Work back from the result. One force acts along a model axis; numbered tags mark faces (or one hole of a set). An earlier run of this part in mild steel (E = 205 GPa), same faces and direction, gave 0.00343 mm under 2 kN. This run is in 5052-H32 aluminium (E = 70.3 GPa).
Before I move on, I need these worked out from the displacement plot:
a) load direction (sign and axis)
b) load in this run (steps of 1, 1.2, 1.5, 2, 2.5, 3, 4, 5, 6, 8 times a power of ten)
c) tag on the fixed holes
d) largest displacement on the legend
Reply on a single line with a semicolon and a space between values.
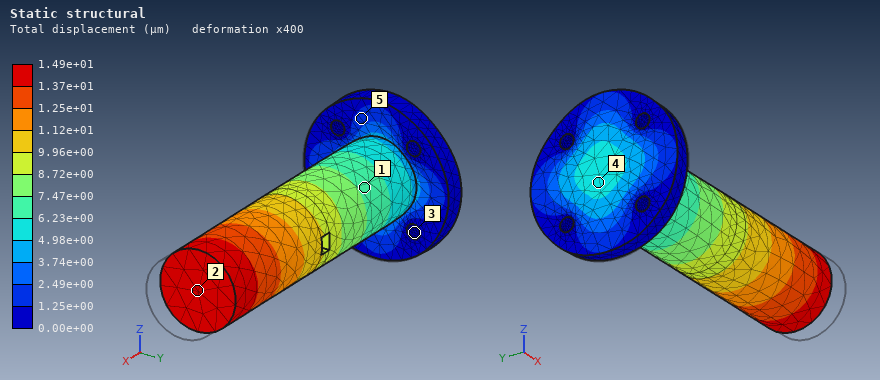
-X; 3 kN; 3; 1.49e+01 µm
